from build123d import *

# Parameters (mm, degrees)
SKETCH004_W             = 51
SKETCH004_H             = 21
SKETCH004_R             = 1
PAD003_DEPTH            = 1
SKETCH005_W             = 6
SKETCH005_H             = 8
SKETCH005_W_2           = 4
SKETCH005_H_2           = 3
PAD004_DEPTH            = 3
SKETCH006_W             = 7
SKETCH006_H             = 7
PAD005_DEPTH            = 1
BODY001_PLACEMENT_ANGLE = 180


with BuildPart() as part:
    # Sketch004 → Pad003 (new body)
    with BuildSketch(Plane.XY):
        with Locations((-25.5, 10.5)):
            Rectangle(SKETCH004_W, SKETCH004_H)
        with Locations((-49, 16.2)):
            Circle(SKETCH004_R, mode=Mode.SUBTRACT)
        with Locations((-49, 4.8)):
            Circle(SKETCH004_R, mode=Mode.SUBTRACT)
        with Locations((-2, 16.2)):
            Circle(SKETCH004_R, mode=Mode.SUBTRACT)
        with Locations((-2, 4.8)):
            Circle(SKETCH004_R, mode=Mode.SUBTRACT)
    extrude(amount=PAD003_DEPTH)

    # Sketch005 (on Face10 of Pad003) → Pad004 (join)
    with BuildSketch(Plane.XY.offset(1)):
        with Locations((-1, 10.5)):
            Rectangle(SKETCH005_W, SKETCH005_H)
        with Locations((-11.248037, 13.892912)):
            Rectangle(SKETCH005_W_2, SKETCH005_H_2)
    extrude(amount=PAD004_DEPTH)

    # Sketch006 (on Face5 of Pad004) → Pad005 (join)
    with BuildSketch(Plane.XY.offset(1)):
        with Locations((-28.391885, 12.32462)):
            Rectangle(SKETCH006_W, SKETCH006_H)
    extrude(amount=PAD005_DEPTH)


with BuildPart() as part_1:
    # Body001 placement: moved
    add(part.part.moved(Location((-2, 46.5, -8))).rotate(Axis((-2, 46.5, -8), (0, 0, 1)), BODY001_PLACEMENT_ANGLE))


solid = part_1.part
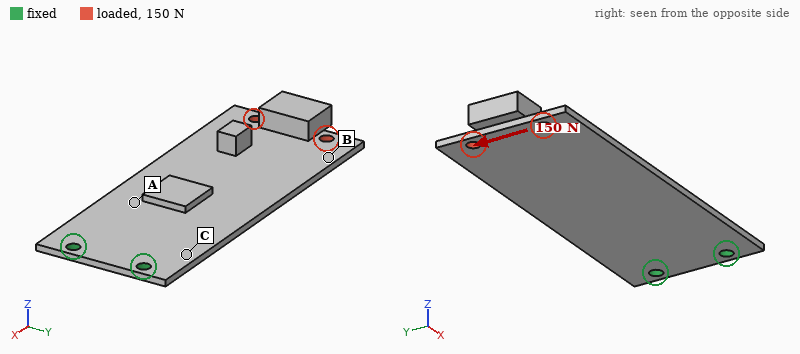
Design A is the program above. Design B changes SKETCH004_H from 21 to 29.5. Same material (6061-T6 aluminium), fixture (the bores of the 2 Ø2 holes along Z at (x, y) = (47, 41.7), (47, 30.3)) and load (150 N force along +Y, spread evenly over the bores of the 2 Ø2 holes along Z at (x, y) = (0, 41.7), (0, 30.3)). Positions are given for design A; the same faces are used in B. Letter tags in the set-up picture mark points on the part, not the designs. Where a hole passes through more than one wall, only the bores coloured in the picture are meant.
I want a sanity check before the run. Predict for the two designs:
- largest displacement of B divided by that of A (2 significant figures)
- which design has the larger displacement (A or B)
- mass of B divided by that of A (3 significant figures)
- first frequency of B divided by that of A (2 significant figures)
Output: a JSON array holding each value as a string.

["0.73", "A", "1.34", "1.0"]
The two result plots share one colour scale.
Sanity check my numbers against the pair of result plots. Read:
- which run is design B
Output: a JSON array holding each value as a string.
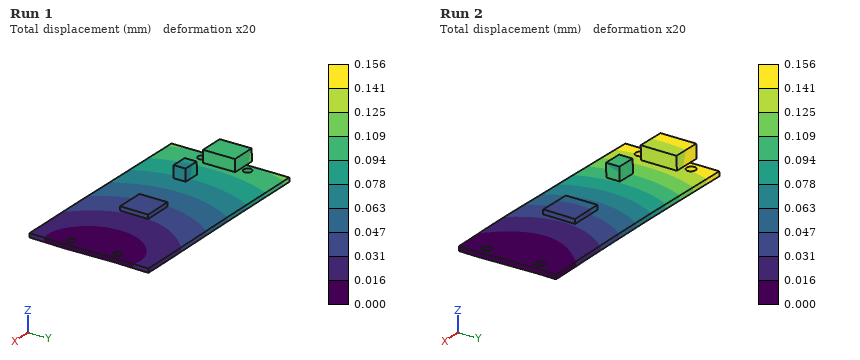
["Run 1"]
